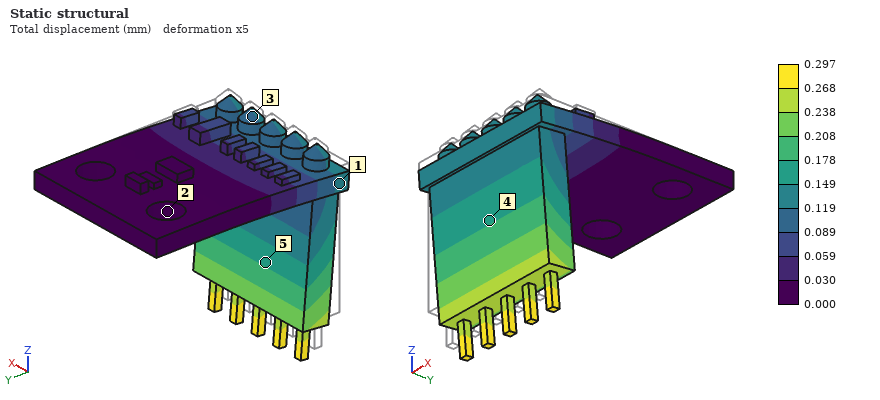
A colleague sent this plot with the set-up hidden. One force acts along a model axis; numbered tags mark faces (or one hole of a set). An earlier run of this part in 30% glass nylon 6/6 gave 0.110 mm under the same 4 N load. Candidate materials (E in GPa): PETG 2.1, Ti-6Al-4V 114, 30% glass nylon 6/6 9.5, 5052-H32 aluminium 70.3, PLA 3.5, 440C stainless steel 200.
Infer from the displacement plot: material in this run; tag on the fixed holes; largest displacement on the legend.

PLA
2
0.297 mm
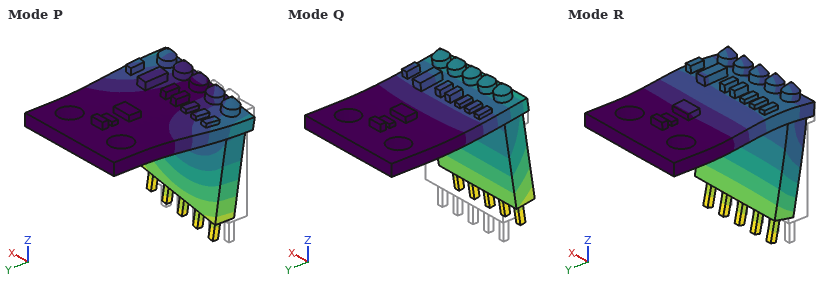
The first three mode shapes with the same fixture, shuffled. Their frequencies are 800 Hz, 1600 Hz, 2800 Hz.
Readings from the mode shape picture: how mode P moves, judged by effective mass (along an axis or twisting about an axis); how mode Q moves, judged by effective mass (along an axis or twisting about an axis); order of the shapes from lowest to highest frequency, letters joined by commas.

along X
along Z
Q, P, R
